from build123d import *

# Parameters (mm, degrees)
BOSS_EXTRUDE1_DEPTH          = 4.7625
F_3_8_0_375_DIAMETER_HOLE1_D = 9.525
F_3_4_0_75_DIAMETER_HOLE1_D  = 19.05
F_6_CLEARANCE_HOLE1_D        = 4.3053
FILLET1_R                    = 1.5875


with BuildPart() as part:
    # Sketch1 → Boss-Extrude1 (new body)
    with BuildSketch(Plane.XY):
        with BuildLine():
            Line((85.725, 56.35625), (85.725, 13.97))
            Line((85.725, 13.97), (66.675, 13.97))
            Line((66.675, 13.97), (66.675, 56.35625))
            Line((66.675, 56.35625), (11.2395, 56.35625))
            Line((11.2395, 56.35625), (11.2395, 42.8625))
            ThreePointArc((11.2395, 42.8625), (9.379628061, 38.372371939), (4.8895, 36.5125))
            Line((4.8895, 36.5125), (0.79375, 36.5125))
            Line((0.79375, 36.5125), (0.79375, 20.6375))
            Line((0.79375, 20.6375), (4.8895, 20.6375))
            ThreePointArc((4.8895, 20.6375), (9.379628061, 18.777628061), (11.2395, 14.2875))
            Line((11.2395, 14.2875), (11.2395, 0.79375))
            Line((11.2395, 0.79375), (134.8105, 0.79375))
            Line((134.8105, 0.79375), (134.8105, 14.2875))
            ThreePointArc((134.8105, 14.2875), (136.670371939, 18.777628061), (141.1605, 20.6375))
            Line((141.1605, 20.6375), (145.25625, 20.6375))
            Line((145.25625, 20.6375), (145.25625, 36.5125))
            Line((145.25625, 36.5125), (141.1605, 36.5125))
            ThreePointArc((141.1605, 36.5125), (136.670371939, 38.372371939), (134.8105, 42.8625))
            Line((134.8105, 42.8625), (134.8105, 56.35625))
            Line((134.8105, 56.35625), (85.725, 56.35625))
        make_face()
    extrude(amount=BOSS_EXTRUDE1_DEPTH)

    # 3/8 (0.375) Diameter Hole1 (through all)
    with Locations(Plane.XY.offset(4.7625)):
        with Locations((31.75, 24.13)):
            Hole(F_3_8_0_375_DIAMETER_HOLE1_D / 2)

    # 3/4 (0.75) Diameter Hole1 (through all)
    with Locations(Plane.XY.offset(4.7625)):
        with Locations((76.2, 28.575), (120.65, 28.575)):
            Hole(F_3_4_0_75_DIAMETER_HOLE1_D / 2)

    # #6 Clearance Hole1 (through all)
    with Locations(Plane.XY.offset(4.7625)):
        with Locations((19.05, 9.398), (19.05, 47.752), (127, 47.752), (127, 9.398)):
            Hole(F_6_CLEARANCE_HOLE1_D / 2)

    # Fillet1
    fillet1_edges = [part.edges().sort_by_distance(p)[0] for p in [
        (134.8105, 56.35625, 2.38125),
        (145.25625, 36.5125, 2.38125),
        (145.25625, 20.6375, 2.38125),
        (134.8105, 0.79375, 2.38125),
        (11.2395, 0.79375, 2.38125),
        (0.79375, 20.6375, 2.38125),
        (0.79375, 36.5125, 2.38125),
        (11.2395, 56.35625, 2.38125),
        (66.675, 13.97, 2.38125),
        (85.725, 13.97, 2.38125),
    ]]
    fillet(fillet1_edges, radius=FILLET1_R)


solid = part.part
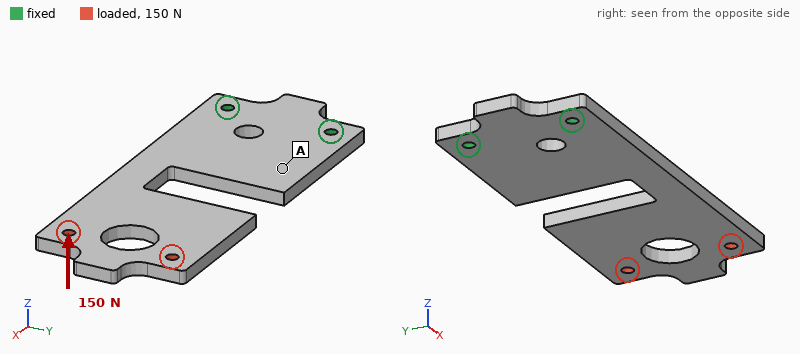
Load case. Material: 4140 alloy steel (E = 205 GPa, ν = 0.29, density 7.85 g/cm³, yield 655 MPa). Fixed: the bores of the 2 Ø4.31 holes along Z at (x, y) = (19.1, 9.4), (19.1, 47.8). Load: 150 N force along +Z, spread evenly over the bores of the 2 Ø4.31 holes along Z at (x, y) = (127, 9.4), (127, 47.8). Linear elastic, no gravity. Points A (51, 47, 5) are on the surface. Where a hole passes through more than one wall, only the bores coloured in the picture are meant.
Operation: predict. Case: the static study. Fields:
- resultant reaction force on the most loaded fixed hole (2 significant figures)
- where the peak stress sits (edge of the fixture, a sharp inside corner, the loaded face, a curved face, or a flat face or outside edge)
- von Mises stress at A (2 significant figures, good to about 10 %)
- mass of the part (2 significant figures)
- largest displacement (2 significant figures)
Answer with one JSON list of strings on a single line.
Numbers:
["78 N", "a curved face", "38 MPa", "220 g", "1.6 mm"]
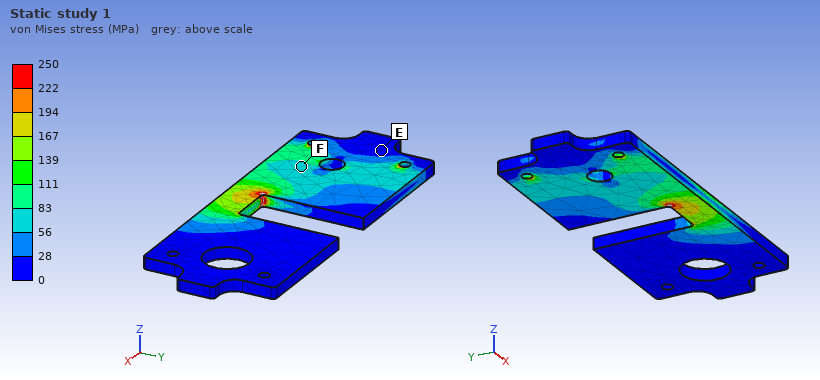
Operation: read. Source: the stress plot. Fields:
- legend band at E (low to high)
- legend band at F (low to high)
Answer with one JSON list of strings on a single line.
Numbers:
["0 to 28 MPa", "56 to 83 MPa"]
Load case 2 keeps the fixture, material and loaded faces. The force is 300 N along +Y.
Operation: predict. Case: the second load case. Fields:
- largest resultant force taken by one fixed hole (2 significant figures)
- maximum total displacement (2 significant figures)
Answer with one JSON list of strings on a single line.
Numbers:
["850 N", "0.22 mm"]
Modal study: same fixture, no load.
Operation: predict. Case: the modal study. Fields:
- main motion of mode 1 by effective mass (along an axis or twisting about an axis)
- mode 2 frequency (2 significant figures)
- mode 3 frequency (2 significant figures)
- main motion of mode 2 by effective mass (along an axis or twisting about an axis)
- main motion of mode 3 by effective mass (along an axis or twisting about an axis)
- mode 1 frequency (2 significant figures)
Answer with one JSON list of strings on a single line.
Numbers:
["along Z", "740 Hz", "790 Hz", "twisting about X", "along Y", "220 Hz"]
